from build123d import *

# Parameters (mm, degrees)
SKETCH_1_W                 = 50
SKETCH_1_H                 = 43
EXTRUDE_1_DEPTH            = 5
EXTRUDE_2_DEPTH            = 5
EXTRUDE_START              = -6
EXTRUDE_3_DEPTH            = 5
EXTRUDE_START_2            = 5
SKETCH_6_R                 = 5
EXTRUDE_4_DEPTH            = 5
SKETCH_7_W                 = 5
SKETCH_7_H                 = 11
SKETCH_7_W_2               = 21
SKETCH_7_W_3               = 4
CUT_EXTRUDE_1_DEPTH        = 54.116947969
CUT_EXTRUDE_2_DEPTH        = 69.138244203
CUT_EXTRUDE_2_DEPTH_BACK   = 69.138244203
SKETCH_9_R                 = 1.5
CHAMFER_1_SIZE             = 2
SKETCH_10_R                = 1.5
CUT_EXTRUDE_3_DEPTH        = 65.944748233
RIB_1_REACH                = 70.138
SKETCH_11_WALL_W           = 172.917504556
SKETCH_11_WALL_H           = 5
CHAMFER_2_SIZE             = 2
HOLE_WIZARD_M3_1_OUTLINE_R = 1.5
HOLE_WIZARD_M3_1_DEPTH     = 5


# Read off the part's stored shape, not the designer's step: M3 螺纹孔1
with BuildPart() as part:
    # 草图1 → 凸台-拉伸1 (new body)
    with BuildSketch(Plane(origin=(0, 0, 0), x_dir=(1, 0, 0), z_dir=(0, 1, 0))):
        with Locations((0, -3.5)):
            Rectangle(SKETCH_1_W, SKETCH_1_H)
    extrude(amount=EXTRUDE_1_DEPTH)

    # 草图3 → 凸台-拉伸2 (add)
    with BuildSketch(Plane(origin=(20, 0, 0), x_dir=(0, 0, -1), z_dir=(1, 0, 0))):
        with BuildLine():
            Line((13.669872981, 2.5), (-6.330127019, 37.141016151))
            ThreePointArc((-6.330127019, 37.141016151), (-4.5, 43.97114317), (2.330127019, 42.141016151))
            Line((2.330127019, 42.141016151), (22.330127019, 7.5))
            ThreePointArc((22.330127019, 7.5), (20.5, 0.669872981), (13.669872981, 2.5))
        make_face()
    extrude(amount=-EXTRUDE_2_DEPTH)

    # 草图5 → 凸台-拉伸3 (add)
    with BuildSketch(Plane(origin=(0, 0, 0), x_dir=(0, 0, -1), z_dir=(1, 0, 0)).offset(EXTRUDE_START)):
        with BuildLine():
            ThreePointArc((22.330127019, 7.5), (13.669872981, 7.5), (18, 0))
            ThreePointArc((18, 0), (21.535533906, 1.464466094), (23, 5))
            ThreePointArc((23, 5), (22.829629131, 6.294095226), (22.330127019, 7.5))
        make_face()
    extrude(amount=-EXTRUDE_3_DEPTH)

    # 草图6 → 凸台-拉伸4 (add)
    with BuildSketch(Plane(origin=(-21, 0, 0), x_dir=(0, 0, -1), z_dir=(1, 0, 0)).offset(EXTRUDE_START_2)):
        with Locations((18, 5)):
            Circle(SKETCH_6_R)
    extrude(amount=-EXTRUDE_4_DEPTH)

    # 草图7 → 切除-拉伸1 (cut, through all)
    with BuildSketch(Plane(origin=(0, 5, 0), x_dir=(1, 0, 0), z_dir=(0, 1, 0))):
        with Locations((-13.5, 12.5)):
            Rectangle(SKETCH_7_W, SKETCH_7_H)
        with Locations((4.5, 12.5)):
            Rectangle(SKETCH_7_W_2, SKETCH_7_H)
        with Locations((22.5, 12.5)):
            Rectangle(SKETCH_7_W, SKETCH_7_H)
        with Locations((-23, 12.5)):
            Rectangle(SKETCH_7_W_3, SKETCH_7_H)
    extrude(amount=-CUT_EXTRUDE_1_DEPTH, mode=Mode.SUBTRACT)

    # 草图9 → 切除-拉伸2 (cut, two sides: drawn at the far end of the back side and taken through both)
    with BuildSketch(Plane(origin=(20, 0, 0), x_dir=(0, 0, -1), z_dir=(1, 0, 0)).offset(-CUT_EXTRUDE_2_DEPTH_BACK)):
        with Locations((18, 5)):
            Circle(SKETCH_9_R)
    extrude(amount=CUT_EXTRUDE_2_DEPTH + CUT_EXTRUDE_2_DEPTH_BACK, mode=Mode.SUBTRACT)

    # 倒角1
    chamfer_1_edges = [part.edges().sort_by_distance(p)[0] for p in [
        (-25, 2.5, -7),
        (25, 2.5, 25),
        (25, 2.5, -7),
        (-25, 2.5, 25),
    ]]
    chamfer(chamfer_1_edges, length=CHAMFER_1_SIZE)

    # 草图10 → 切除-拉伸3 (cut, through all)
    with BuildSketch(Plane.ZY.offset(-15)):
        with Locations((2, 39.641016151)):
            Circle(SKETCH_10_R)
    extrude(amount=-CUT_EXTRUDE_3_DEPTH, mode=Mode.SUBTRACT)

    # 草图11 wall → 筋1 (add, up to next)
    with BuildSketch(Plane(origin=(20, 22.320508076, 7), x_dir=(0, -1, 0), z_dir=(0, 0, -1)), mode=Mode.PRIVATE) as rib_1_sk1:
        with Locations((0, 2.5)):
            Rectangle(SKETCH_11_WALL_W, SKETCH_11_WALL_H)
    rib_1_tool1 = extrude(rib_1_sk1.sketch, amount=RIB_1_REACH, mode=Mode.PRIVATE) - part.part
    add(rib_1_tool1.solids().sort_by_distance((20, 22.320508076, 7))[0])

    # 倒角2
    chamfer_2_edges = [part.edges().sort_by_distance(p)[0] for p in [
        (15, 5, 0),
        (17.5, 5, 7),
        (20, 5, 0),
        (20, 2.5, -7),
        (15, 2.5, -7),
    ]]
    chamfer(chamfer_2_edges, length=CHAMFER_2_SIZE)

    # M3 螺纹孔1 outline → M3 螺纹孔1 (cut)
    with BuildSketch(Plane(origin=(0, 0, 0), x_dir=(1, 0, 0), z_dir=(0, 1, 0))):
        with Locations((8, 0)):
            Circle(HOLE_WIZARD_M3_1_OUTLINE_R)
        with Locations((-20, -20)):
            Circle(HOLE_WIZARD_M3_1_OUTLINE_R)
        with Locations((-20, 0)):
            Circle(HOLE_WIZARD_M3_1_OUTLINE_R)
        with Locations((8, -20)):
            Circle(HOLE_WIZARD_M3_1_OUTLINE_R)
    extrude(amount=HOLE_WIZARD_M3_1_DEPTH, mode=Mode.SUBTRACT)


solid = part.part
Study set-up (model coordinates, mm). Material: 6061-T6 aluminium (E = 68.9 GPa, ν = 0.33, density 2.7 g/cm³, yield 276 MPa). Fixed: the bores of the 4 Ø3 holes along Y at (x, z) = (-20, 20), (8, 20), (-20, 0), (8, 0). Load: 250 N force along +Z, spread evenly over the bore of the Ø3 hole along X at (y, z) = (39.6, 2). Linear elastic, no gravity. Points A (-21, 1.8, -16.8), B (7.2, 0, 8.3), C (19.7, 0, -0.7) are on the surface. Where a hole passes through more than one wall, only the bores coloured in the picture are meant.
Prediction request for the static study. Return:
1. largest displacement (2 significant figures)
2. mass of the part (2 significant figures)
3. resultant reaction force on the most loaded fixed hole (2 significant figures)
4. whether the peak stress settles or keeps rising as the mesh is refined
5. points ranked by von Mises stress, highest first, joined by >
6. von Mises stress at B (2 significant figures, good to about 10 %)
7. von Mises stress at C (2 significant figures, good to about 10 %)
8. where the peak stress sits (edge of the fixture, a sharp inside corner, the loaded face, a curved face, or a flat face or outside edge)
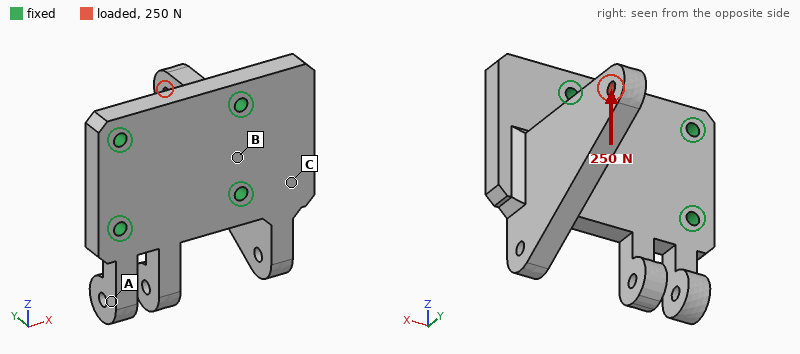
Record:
0.11 mm
35 g
400 N
keeps rising
C > B > A
14 MPa
25 MPa
edge of the fixture
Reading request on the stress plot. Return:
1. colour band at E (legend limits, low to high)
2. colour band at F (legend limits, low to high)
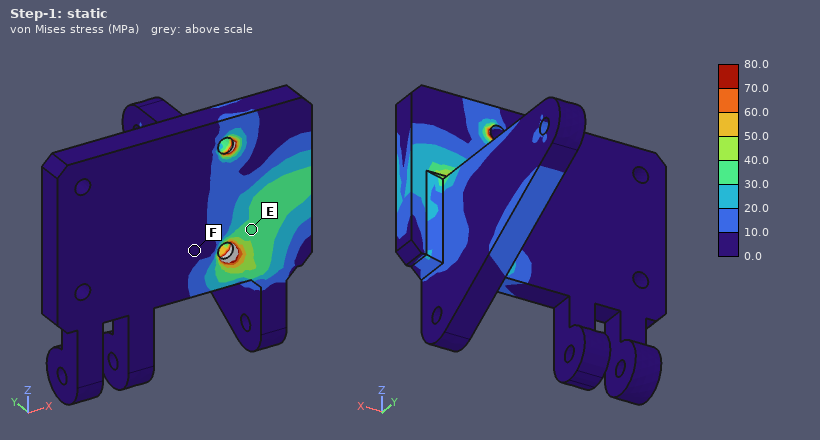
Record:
30.0 to 40.0 MPa
0.0 to 10.0 MPa
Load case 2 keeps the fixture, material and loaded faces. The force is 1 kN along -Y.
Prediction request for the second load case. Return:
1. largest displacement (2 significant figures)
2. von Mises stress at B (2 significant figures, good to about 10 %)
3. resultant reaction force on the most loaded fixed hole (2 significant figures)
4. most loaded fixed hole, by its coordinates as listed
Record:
0.12 mm
27 MPa
910 N
(8, 0)
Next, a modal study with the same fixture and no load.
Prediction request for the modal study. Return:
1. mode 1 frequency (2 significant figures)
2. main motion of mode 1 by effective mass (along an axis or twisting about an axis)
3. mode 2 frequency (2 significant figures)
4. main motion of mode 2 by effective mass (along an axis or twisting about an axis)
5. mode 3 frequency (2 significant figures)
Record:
2400 Hz
along X
4200 Hz
along Z
6900 Hz
